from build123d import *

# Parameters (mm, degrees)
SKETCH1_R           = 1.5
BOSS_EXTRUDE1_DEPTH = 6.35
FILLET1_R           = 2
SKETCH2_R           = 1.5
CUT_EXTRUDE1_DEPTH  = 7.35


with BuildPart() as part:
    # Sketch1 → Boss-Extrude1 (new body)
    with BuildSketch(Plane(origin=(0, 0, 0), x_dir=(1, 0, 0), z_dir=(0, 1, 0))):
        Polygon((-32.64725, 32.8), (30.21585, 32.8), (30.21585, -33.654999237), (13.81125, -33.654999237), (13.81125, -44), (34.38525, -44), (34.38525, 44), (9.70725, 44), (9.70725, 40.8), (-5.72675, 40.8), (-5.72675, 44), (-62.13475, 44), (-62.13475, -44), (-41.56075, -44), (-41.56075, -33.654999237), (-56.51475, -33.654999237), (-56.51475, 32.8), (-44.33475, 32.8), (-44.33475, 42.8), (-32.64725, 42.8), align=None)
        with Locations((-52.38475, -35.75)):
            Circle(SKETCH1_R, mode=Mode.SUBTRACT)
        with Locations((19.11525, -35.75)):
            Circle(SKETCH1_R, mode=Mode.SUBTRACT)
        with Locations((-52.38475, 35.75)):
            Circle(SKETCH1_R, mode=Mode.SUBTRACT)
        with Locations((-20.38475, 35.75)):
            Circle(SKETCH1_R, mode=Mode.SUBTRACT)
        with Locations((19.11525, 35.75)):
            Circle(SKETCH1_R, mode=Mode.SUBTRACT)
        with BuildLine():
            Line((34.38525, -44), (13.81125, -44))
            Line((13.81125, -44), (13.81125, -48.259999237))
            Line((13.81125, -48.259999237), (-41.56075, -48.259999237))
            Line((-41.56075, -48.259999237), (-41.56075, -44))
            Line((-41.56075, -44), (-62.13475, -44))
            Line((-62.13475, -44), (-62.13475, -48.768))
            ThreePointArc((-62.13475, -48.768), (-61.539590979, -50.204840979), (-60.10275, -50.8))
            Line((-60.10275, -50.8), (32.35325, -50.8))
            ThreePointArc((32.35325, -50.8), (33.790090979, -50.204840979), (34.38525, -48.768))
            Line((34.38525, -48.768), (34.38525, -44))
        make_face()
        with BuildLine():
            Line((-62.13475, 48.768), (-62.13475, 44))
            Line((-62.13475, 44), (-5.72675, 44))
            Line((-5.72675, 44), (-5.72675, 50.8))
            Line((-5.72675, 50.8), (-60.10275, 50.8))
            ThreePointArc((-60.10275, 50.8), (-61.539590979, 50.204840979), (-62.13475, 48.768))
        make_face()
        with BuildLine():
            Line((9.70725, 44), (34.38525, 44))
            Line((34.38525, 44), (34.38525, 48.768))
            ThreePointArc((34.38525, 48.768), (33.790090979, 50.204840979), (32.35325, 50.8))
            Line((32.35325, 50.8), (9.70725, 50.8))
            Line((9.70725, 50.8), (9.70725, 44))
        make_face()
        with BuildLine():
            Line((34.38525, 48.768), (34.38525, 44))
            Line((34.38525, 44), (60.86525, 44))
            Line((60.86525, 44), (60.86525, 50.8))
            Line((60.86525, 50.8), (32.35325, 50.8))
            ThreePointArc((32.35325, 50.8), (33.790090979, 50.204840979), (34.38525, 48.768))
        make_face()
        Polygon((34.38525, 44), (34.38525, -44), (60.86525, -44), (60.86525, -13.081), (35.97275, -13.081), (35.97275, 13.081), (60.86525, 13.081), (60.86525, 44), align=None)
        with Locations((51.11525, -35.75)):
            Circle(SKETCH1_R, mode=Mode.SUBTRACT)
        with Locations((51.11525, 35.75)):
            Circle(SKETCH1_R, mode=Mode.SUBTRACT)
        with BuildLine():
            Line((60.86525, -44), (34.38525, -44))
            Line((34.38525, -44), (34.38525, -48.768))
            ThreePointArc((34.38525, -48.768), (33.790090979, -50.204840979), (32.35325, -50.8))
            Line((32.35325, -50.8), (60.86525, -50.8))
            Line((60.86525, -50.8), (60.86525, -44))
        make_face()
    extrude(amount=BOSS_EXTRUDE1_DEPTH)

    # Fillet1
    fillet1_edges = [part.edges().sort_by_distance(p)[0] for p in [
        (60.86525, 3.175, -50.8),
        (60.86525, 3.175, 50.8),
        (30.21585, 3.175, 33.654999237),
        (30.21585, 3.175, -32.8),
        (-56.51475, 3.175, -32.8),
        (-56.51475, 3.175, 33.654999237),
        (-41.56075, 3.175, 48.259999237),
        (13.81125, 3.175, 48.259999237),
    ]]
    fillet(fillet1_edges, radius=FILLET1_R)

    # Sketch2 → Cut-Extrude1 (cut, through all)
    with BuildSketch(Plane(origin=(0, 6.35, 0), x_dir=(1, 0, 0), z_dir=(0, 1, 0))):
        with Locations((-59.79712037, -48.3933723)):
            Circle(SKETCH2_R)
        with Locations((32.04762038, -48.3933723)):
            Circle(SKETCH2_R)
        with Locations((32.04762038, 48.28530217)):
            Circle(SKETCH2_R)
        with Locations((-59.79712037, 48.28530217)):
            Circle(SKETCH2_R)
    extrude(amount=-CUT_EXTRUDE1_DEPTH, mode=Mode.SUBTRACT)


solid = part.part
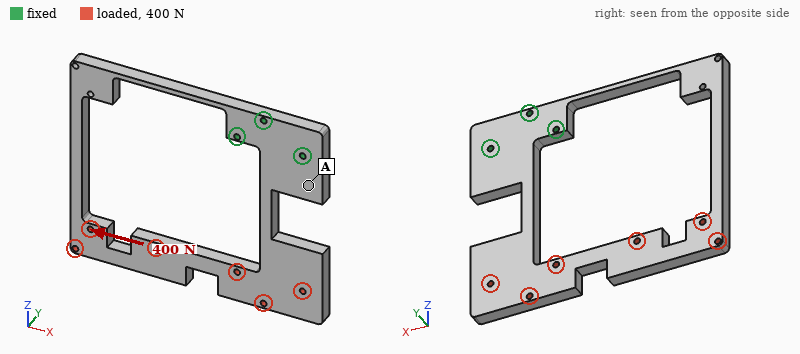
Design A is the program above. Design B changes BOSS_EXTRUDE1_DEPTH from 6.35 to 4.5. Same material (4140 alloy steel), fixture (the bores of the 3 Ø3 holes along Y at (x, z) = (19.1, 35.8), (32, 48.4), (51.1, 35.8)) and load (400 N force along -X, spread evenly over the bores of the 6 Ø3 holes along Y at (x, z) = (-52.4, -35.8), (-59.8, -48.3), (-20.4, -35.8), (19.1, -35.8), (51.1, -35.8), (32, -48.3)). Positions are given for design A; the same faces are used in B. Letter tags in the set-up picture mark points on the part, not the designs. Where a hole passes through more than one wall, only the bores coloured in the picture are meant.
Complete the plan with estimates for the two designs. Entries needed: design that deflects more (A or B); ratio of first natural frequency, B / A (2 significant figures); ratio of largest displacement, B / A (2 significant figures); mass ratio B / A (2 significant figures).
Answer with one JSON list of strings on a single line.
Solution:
["B", "0.75", "1.4", "0.71"]
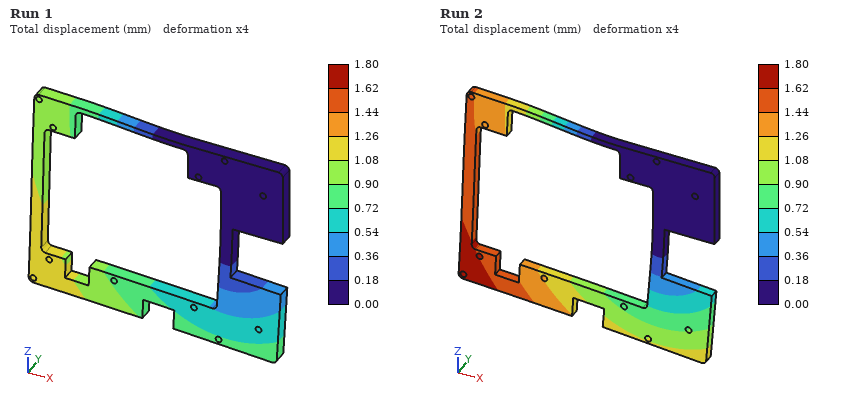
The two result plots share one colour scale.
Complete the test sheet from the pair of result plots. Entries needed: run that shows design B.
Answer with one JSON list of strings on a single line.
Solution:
["Run 2"]
